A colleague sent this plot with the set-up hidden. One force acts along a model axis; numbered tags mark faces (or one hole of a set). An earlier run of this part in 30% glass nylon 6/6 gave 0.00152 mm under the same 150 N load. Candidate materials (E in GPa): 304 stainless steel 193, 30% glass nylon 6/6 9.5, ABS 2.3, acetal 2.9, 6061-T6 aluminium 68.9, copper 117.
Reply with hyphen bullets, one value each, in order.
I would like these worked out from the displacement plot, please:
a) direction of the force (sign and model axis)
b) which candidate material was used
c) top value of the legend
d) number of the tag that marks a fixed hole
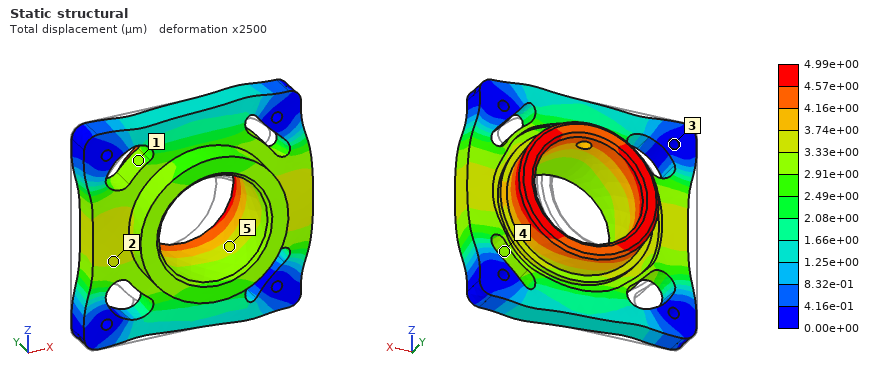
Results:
- +X
- acetal
- 4.99e+00 µm
- 3
